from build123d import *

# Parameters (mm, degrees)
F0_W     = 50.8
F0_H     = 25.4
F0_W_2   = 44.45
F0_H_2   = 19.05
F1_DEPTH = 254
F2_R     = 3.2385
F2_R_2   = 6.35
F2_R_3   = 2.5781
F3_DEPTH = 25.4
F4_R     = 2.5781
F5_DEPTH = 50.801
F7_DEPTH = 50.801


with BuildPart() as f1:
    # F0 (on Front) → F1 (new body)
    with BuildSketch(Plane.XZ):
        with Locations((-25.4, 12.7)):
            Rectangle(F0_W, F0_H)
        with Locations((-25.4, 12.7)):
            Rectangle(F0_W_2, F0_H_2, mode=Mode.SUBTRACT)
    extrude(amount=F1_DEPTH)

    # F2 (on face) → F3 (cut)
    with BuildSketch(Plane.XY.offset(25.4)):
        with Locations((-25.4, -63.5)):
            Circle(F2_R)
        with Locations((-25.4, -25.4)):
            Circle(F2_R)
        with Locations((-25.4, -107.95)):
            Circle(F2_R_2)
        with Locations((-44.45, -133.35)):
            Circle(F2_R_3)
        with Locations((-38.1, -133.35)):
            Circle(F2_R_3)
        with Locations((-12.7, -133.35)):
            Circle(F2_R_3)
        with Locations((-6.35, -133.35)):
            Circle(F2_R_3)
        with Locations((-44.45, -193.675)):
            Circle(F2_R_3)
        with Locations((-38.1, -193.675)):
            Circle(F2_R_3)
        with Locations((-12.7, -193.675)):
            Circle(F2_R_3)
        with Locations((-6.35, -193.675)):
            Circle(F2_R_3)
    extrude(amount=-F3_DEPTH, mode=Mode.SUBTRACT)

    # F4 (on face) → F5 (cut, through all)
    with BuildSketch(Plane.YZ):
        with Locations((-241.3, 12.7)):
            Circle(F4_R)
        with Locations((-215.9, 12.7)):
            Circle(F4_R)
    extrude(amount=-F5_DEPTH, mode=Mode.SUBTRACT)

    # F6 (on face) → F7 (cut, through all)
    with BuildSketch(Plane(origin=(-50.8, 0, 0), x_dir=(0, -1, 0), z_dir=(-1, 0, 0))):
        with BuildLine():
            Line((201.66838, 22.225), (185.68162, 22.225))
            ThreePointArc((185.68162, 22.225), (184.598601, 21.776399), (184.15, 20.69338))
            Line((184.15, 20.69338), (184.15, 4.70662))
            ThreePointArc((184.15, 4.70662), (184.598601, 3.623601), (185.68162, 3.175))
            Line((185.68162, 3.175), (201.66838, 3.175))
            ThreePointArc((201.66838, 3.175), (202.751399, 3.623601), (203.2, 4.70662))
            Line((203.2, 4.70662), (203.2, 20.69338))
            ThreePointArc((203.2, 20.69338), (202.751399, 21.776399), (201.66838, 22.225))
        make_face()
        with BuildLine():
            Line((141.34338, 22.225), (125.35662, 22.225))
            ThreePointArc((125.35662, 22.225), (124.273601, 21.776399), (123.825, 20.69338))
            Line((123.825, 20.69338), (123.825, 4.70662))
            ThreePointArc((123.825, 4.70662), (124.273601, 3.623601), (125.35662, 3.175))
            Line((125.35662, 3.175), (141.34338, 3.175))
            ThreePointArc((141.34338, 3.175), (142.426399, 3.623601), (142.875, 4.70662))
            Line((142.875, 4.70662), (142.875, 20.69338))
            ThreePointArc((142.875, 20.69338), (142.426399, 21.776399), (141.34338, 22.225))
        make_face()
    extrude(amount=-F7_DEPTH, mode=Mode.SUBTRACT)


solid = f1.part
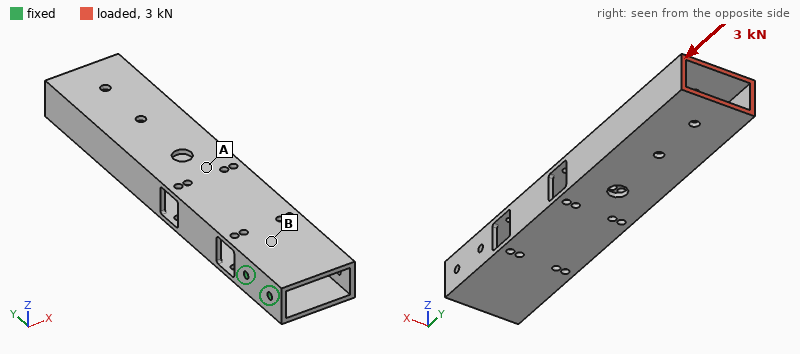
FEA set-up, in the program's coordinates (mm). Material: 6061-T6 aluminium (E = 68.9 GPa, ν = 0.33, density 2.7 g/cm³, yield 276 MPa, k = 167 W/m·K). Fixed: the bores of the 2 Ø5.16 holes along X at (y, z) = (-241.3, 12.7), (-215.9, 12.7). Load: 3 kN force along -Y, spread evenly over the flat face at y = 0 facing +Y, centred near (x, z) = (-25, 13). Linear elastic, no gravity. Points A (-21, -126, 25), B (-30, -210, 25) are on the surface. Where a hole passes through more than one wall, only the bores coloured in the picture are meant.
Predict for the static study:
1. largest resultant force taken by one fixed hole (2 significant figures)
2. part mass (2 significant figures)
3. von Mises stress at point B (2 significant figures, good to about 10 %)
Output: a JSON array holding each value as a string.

["2.8 kN", "280 g", "24 MPa"]
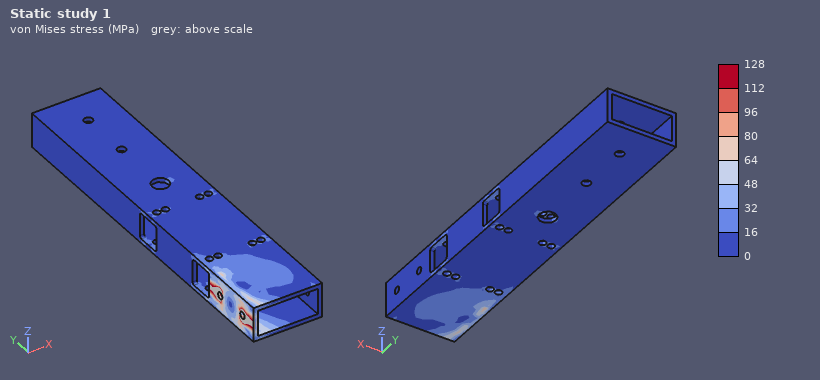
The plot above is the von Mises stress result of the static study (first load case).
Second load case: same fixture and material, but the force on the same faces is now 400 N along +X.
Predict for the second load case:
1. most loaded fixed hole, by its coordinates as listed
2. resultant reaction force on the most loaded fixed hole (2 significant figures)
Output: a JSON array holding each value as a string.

["(-215.9, 12.7)", "3.2 kN"]
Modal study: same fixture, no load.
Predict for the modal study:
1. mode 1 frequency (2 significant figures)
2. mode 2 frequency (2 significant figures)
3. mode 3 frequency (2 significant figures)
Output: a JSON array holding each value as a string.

["270 Hz", "280 Hz", "610 Hz"]
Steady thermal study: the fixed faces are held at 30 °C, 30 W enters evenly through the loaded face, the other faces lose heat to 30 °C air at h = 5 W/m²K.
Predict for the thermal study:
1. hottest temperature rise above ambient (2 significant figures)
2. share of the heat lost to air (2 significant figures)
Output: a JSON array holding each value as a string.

["82 K", "45 %"]
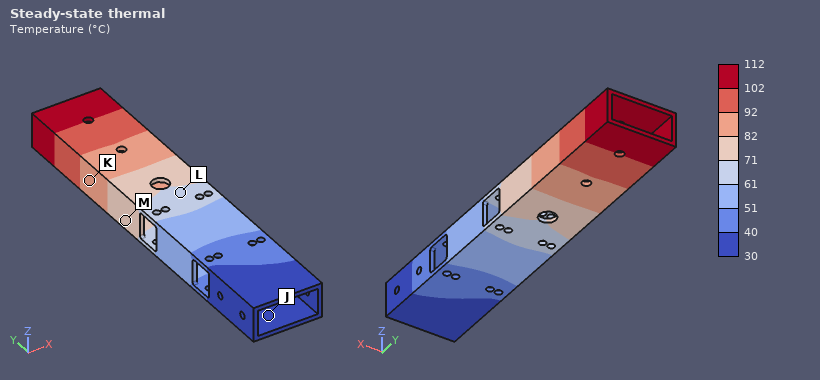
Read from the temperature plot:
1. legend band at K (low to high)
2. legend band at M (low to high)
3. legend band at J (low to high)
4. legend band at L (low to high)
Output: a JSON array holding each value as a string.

["82 to 92 °C", "71 to 82 °C", "30 to 40 °C", "61 to 71 °C"]
